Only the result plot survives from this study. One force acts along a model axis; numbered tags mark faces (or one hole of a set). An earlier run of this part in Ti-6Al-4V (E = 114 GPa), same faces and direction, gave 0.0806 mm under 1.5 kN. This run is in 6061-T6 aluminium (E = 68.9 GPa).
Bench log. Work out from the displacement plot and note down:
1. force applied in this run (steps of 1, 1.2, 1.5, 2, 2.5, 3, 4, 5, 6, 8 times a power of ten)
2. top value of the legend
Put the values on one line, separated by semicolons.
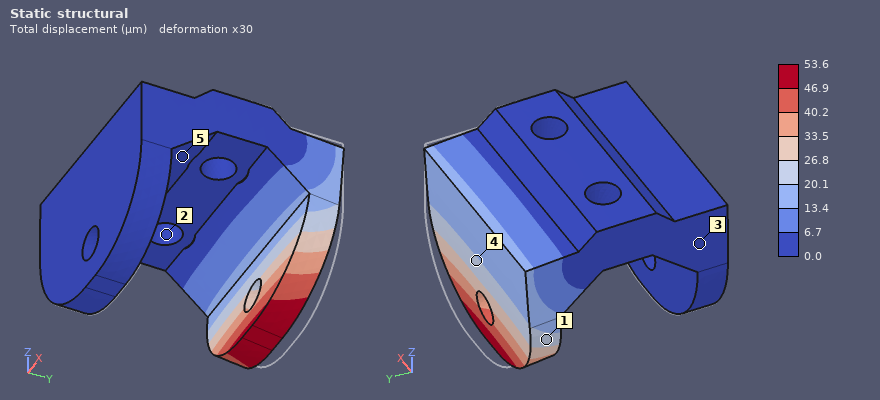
600 N; 53.6 µm
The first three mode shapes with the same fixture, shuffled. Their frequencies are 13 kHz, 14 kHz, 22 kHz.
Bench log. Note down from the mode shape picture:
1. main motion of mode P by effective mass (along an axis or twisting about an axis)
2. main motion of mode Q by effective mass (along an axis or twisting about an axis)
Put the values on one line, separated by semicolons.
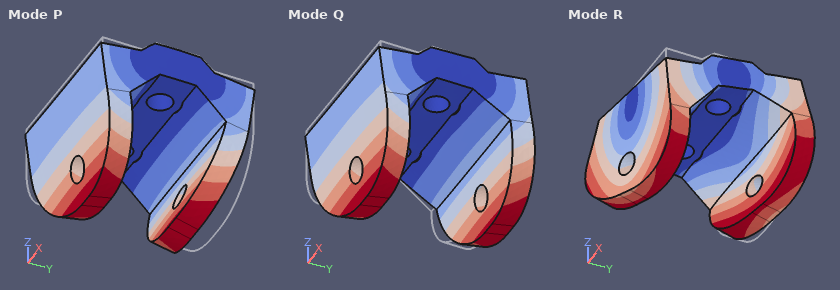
along Z; along Y
